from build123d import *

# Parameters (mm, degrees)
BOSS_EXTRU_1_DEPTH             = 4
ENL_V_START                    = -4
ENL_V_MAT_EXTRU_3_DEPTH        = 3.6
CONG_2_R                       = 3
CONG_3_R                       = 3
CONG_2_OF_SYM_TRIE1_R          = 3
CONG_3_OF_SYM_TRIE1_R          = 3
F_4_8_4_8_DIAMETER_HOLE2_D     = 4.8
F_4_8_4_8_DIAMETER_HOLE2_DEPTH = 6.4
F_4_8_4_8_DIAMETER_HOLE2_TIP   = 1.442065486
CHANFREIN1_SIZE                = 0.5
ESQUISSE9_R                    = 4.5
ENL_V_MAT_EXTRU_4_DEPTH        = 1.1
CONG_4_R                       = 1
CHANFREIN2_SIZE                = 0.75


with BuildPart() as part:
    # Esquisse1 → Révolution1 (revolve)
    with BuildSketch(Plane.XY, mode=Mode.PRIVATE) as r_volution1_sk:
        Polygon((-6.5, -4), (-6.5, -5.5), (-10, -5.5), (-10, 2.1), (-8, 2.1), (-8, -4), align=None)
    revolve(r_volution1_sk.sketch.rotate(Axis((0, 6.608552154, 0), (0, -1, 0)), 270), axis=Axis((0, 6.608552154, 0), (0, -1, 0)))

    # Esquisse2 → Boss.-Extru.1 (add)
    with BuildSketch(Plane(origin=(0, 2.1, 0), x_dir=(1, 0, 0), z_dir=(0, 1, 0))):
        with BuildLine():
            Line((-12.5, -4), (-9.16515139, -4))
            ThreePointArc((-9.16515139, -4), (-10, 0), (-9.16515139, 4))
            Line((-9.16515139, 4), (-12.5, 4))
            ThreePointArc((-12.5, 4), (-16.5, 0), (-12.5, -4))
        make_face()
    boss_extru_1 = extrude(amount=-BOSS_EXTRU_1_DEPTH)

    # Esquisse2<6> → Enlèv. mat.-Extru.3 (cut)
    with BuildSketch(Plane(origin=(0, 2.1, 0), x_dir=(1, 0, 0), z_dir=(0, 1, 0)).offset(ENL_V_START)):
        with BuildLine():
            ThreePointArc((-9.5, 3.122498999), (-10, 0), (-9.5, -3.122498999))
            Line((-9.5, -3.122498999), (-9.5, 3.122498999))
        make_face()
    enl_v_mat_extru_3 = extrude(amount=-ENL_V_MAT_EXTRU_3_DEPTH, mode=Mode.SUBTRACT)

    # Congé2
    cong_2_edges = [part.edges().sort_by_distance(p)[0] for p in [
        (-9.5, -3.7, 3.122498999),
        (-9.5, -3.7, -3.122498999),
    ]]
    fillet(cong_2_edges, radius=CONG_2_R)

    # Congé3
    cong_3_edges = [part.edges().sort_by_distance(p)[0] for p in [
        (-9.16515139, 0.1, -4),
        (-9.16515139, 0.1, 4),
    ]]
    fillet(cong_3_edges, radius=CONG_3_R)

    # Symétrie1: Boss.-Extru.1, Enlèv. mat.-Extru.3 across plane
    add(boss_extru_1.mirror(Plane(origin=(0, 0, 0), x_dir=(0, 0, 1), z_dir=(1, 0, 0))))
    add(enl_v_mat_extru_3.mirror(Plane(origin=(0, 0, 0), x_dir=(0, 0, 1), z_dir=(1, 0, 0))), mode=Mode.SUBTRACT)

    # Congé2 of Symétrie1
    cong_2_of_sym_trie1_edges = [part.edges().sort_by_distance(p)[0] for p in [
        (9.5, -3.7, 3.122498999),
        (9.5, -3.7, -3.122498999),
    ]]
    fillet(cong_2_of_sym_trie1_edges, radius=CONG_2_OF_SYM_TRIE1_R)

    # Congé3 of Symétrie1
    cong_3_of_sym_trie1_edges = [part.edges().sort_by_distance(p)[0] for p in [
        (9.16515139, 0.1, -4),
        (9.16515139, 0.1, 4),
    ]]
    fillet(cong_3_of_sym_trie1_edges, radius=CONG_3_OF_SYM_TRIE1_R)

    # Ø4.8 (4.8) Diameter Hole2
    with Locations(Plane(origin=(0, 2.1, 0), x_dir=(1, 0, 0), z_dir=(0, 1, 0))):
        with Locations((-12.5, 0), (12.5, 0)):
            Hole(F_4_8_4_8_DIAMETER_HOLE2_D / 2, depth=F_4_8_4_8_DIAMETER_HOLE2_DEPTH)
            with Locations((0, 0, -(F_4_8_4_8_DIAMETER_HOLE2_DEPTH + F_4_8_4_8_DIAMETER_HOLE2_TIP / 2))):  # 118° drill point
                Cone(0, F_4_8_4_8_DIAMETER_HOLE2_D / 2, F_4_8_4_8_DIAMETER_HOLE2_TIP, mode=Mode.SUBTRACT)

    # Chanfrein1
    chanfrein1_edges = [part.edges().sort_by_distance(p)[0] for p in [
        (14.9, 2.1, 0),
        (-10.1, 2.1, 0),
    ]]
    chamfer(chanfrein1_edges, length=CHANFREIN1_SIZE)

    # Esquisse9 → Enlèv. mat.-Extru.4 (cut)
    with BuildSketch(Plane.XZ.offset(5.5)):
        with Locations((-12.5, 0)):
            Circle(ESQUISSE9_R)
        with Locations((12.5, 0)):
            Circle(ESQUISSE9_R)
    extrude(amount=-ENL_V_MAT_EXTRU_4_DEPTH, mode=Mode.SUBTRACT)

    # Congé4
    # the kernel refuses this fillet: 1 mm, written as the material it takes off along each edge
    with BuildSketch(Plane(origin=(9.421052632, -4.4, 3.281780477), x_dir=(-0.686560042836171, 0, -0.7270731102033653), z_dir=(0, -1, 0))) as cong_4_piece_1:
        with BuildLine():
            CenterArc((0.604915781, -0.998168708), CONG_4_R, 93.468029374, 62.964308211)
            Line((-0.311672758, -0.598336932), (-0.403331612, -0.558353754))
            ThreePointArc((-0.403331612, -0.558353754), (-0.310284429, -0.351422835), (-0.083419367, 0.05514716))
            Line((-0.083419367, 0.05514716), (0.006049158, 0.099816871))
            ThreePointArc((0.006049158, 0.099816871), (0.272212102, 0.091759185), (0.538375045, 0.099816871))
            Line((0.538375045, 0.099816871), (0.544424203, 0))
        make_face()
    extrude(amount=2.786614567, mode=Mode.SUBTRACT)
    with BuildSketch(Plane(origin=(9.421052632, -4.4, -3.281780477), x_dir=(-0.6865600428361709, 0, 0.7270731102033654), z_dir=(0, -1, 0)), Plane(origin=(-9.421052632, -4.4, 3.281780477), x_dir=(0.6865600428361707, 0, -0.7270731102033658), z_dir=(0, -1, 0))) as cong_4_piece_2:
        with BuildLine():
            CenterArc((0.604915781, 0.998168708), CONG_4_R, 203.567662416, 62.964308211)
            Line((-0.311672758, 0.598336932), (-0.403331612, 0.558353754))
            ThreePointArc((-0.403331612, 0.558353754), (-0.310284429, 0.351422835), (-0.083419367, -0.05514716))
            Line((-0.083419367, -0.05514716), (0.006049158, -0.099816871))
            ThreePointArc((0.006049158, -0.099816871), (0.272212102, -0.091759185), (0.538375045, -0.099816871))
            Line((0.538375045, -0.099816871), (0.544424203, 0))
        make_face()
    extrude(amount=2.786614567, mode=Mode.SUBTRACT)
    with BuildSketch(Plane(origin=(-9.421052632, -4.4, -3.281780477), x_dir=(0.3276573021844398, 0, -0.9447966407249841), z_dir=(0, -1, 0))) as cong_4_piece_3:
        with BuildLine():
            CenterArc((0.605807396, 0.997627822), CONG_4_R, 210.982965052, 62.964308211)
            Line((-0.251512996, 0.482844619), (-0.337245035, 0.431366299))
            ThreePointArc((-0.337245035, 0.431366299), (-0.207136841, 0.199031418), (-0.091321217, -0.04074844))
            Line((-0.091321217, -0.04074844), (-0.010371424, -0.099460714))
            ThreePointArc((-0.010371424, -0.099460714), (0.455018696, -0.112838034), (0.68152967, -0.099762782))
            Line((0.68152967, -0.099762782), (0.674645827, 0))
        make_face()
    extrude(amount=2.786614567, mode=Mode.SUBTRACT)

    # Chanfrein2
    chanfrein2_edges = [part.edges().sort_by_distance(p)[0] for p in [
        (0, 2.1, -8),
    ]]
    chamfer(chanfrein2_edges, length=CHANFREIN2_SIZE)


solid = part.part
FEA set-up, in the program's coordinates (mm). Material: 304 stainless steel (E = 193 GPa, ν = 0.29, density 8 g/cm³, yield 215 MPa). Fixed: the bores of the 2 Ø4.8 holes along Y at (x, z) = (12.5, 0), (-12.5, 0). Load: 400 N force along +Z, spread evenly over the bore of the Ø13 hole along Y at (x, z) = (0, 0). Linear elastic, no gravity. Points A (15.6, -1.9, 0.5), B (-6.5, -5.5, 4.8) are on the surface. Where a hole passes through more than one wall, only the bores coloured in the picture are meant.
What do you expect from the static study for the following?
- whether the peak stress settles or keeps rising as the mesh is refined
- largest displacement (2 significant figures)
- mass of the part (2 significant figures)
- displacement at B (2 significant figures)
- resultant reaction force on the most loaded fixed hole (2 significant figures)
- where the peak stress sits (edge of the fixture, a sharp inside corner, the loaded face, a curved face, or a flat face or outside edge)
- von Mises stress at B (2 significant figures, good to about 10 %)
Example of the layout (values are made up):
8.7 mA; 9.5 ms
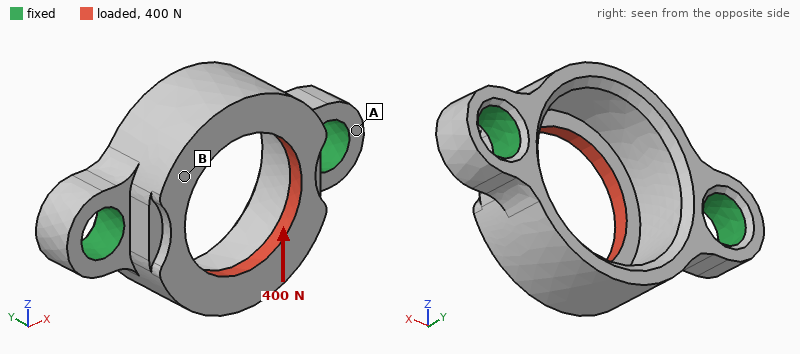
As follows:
keeps rising; 4.6 µm; 9.2 g; 2.6 µm; 200 N; edge of the fixture; 14 MPa
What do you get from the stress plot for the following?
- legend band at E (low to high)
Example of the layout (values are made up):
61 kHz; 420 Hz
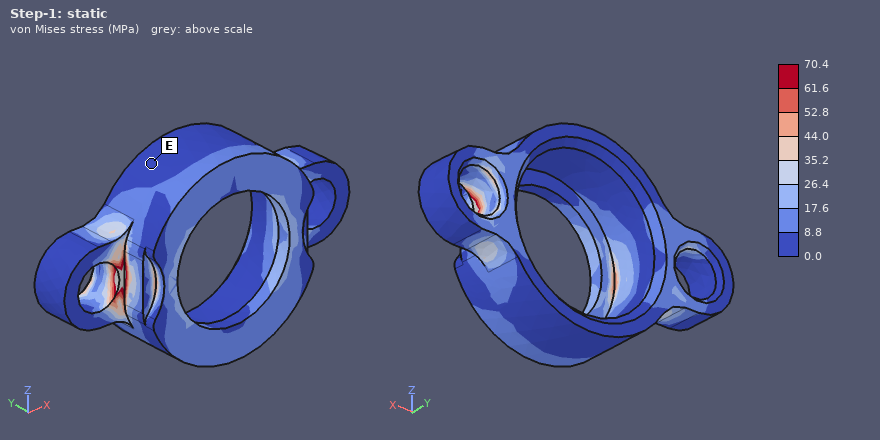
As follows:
0.0 to 8.8 MPa
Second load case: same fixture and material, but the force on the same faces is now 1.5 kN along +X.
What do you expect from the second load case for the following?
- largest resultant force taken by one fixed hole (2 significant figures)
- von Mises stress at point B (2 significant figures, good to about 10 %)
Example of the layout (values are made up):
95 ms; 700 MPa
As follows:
800 N; 43 MPa
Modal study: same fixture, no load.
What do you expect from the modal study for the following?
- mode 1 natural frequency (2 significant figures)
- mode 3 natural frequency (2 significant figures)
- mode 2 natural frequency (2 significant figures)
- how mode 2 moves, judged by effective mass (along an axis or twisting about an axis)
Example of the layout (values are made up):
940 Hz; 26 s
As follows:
20 kHz; 35 kHz; 26 kHz; along Y
